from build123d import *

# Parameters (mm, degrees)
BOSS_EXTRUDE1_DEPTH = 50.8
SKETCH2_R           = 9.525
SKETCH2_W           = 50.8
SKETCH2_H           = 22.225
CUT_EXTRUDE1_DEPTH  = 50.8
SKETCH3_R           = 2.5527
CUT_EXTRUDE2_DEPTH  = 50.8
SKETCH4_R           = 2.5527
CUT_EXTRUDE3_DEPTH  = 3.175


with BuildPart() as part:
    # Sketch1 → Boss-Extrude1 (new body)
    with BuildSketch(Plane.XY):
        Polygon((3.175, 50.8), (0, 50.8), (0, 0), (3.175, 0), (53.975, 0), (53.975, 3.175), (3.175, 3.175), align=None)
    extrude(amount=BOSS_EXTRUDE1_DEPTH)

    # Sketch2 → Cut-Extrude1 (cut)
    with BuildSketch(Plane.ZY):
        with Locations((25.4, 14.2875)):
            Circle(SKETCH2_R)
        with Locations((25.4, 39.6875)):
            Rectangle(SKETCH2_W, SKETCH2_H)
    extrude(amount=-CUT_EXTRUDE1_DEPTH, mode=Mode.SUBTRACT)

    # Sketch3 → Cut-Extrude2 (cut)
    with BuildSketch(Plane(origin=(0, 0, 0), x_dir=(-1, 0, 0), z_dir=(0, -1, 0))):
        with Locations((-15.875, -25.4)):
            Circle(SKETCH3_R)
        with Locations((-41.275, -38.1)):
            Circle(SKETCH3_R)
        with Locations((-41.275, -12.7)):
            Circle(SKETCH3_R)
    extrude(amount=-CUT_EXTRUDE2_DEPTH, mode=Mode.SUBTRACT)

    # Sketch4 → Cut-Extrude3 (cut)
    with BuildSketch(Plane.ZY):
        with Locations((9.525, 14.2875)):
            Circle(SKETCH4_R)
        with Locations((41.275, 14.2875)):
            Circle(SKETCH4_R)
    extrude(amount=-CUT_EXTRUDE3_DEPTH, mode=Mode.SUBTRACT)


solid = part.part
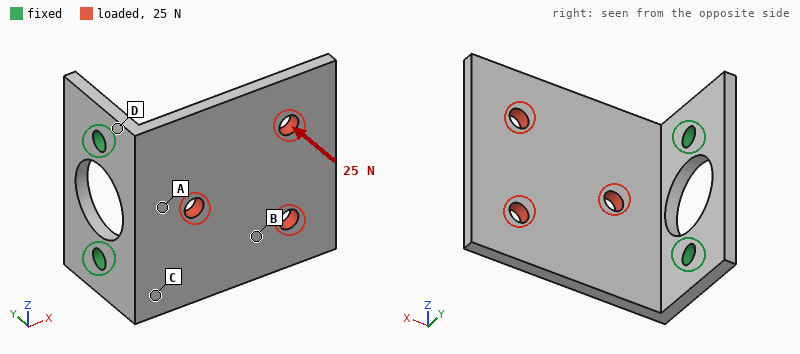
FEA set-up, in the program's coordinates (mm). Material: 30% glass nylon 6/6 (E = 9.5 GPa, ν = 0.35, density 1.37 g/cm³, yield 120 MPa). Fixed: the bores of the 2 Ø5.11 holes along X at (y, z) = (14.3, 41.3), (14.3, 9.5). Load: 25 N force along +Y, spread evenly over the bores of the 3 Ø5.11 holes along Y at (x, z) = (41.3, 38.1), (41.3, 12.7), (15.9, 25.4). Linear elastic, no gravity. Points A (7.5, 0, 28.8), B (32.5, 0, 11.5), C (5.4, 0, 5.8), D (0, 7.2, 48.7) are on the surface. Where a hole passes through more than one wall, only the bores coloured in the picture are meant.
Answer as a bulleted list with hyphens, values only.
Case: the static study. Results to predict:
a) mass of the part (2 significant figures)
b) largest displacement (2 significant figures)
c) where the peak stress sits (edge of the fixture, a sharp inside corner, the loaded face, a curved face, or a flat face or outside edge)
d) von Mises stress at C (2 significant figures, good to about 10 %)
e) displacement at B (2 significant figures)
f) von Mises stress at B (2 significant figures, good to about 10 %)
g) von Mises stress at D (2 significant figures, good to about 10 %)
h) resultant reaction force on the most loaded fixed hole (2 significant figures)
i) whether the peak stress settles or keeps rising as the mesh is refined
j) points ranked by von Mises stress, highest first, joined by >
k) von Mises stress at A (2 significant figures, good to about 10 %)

- 16 g
- 0.90 mm
- edge of the fixture
- 8.2 MPa
- 0.48 mm
- 1.9 MPa
- 11 MPa
- 13 N
- keeps rising
- D > C > A > B
- 5.7 MPa
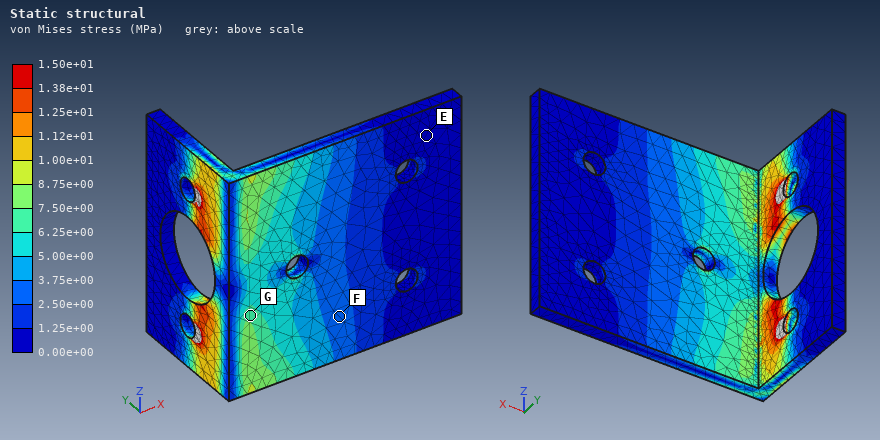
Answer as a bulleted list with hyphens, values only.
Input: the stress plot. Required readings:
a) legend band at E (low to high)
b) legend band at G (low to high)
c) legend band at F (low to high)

- 0.00e+00 to 1.25e+00 MPa
- 6.25e+00 to 7.50e+00 MPa
- 2.50e+00 to 3.75e+00 MPa
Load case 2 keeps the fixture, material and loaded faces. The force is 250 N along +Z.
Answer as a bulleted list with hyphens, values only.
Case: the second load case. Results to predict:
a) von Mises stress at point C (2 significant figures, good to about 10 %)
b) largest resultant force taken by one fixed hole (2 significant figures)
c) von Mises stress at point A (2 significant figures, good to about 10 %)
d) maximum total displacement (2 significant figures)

- 15 MPa
- 250 N
- 7.0 MPa
- 0.65 mm
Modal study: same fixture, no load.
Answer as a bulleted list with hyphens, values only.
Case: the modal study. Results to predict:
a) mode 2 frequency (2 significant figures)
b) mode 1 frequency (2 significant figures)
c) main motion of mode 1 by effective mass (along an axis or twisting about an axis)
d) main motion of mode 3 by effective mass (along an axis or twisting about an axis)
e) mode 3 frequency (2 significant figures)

- 1000 Hz
- 340 Hz
- along Y
- along Z
- 1400 Hz
